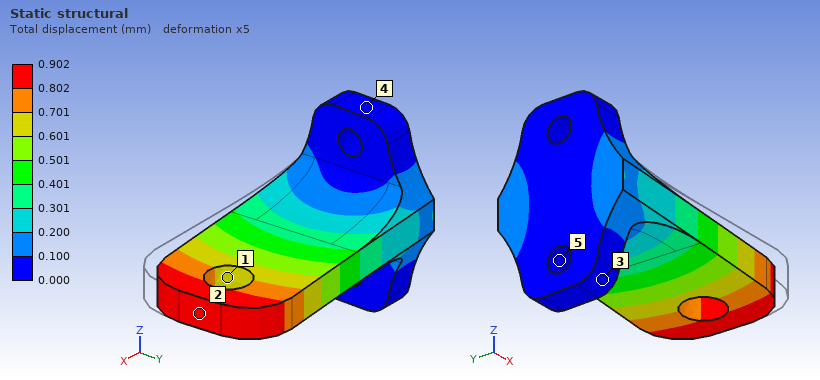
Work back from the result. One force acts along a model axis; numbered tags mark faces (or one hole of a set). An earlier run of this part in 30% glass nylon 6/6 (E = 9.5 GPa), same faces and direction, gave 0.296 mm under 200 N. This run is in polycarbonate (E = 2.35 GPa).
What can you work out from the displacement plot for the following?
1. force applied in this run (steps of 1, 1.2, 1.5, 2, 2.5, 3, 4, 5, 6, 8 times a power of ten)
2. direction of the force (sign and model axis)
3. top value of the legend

150 N
+Y
0.902 mm
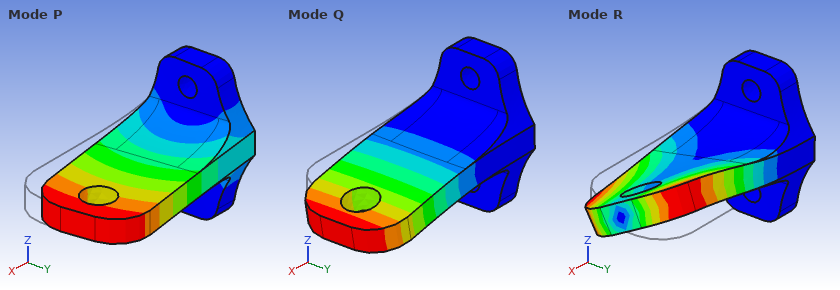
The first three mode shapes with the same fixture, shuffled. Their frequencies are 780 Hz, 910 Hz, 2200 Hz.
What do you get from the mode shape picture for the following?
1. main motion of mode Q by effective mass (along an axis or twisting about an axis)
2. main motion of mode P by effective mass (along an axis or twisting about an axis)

along Z
along Y
